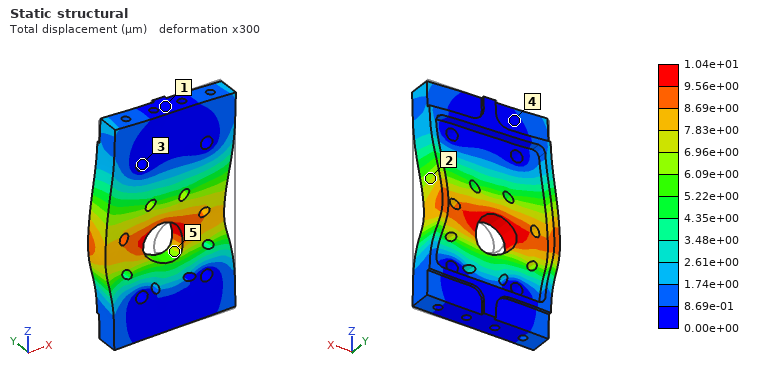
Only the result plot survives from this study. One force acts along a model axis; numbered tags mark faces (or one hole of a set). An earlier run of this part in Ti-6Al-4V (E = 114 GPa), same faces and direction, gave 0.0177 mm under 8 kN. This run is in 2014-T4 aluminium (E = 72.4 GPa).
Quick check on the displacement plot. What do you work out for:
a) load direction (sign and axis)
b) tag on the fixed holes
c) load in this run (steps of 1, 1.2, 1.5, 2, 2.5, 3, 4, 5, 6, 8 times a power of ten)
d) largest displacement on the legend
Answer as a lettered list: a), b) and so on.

a) -X
b) 3
c) 3 kN
d) 1.04e+01 µm
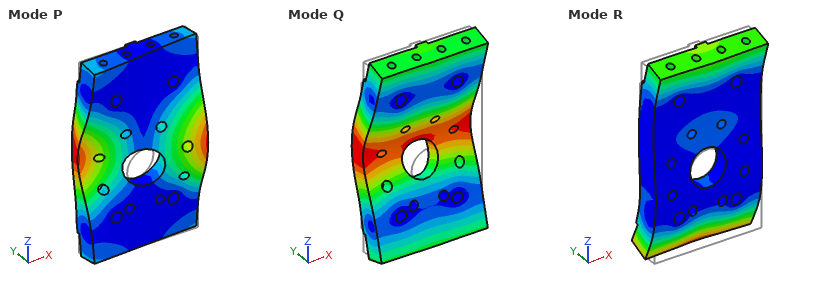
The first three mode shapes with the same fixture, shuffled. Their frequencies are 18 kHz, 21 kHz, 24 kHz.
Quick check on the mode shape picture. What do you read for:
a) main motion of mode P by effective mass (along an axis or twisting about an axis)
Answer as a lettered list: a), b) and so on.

a) twisting about Z
